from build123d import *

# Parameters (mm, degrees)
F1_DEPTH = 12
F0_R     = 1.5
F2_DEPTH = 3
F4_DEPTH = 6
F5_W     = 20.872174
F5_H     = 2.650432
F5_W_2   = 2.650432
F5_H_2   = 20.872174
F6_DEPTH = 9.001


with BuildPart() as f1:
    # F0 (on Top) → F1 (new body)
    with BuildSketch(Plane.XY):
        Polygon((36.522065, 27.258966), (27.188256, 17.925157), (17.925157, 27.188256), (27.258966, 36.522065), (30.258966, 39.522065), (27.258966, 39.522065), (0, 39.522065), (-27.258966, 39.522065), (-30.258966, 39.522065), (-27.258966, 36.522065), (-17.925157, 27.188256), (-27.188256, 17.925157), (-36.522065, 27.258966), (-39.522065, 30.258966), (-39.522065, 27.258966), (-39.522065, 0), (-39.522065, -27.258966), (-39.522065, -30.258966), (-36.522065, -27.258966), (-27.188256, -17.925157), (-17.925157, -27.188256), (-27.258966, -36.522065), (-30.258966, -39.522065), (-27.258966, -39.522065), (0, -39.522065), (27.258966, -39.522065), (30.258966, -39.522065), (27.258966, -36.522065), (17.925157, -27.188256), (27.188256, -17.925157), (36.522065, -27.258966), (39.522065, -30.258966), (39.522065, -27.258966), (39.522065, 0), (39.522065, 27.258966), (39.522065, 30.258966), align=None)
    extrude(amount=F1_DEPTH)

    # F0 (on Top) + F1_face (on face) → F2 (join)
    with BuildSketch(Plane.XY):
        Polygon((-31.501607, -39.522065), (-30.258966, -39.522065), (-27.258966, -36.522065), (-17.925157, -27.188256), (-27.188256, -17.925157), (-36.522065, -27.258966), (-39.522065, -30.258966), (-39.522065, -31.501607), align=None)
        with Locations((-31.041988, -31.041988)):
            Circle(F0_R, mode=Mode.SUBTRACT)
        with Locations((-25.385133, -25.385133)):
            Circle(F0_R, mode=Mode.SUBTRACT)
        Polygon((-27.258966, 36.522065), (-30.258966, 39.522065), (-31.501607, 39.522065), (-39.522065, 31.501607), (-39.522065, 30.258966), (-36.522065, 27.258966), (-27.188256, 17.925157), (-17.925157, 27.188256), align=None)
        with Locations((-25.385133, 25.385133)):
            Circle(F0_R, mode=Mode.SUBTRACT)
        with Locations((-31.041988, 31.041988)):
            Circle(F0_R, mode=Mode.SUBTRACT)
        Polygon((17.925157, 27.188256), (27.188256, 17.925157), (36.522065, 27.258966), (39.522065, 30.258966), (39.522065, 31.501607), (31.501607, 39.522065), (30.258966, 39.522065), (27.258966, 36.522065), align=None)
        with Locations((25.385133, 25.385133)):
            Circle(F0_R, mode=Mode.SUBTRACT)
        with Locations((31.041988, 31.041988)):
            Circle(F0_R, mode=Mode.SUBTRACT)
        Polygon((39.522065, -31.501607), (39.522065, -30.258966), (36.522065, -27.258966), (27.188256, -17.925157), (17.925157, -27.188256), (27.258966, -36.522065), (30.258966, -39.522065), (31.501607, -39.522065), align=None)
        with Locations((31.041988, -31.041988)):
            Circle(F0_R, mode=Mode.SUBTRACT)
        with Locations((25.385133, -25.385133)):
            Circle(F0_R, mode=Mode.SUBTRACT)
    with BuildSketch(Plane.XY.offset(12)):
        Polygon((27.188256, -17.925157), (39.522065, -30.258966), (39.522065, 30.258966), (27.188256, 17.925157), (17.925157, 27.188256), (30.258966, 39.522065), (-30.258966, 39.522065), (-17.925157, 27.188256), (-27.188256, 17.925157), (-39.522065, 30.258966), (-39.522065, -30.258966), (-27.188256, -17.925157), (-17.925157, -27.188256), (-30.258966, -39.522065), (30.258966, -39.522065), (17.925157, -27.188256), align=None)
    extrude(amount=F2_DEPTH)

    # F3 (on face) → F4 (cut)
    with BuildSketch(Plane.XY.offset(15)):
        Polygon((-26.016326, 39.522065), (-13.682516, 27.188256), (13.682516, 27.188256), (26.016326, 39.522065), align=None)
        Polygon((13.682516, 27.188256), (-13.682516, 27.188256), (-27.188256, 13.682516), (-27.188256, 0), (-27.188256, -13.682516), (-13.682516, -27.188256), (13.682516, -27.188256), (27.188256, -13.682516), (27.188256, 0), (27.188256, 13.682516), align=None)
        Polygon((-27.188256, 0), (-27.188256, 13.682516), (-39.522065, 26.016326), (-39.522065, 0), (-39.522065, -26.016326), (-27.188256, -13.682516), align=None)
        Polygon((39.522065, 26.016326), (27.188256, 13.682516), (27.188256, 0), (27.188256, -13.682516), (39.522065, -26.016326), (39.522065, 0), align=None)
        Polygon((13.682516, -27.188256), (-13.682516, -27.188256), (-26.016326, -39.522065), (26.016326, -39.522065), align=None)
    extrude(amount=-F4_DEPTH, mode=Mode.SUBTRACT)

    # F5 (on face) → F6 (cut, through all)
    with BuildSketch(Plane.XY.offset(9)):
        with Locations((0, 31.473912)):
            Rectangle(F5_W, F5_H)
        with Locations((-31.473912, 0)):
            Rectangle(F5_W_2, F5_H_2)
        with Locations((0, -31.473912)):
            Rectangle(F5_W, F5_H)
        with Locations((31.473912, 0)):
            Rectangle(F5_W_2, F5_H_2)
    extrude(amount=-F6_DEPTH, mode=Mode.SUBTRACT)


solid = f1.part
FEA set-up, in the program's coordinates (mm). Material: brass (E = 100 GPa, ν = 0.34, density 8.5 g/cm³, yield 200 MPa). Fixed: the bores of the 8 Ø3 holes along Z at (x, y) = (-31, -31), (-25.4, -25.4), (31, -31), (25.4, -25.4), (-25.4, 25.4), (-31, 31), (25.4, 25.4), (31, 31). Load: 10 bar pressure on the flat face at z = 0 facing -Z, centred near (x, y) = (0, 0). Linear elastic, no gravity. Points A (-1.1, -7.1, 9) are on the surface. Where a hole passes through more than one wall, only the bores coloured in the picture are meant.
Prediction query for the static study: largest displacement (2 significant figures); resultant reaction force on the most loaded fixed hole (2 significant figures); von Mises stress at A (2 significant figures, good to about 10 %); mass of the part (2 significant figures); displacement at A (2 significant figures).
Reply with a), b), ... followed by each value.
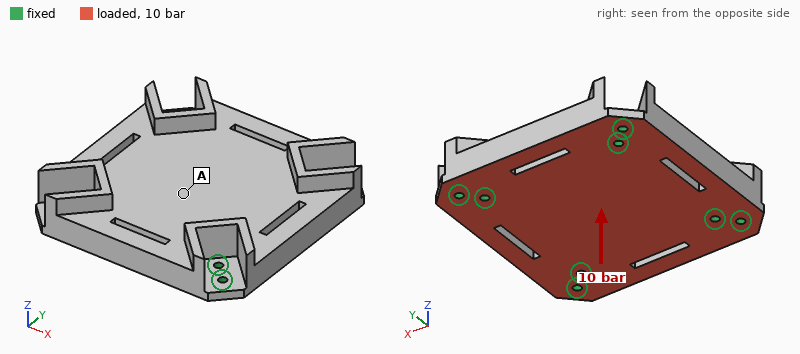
a) 18 µm
b) 1.3 kN
c) 14 MPa
d) 430 g
e) 17 µm
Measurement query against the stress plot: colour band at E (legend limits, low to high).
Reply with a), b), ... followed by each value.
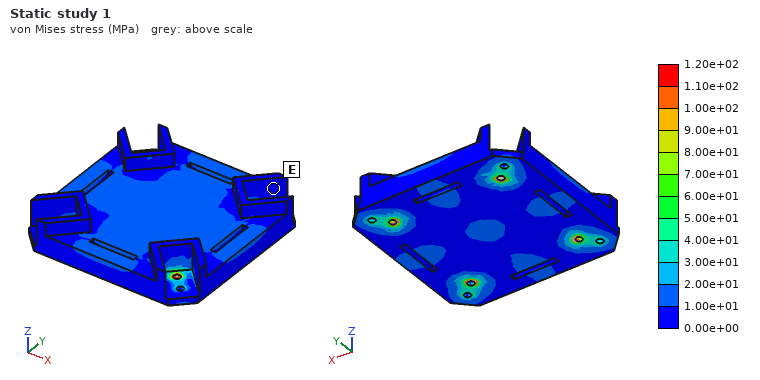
a) 0.00e+00 to 1.00e+01 MPa
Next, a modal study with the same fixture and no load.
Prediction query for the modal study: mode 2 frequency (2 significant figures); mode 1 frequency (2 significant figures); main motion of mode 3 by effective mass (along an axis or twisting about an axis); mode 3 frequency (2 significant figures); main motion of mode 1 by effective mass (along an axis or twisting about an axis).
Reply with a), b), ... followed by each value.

a) 5900 Hz
b) 5000 Hz
c) twisting about X
d) 6200 Hz
e) along Z
